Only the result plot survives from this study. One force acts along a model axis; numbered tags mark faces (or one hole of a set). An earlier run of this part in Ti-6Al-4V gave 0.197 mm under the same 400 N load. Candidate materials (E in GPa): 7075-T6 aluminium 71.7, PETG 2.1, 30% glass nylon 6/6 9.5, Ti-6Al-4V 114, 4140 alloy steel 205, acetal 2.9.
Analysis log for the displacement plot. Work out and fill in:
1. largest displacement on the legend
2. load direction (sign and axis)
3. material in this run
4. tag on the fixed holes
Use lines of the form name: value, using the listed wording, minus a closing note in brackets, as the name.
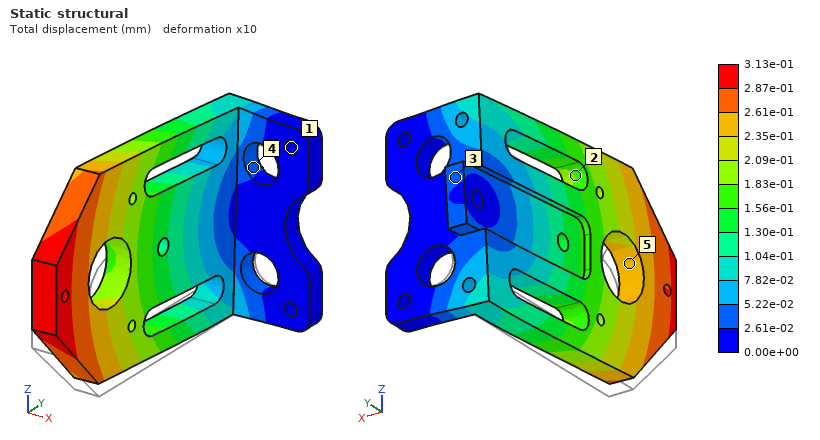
largest displacement on the legend: 3.13e-01 mm
load direction: +Z
material in this run: 7075-T6 aluminium
tag on the fixed holes: 1
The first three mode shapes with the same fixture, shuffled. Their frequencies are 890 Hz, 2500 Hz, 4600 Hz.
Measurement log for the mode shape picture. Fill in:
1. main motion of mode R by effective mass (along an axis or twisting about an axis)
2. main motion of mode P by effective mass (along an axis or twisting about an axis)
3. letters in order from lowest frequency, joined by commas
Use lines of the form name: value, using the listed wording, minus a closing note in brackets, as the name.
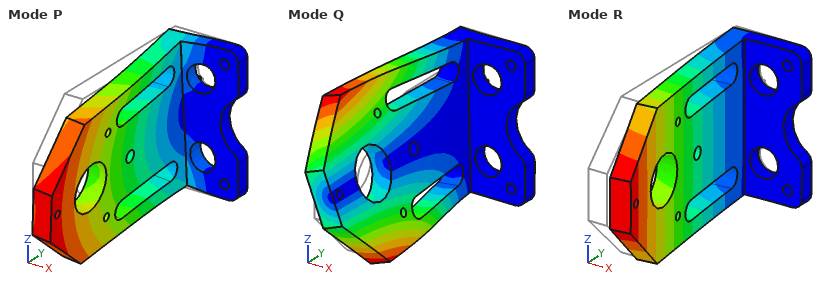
main motion of mode R by effective mass: along X
main motion of mode P by effective mass: along Z
letters in order from lowest frequency, joined by commas: R, P, Q
